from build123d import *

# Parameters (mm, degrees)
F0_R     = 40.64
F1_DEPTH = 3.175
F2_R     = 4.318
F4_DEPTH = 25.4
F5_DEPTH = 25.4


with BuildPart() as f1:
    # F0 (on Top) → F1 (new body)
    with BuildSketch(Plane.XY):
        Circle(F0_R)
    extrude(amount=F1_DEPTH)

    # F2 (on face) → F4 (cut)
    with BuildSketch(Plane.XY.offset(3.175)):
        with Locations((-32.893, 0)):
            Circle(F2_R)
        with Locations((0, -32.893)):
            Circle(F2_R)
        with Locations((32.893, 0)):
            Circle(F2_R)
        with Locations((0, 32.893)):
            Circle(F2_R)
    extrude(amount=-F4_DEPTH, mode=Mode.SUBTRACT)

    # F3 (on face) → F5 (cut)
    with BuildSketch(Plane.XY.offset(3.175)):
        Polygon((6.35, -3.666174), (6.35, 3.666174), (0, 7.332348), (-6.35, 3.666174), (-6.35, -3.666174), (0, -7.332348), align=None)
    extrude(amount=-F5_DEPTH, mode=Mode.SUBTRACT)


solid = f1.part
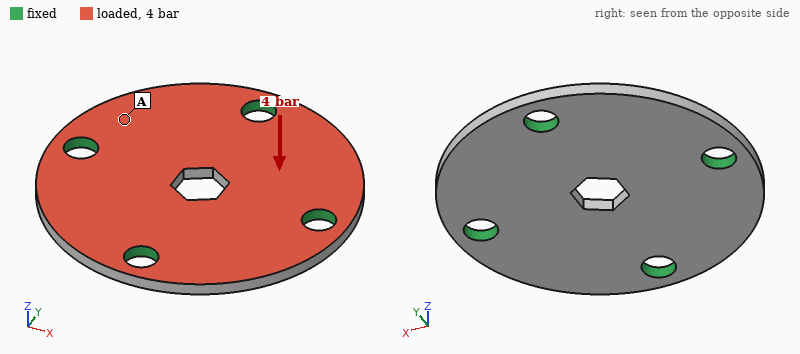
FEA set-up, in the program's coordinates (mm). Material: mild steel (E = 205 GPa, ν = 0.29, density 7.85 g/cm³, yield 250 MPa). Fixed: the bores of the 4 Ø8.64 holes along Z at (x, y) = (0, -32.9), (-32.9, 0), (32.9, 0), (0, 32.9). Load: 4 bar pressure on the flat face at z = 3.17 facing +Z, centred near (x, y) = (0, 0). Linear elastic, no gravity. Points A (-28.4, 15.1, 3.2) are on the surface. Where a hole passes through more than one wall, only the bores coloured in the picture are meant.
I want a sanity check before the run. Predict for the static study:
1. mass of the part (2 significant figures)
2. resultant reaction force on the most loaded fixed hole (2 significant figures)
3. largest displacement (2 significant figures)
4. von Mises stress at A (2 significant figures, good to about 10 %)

120 g
480 N
12 µm
11 MPa
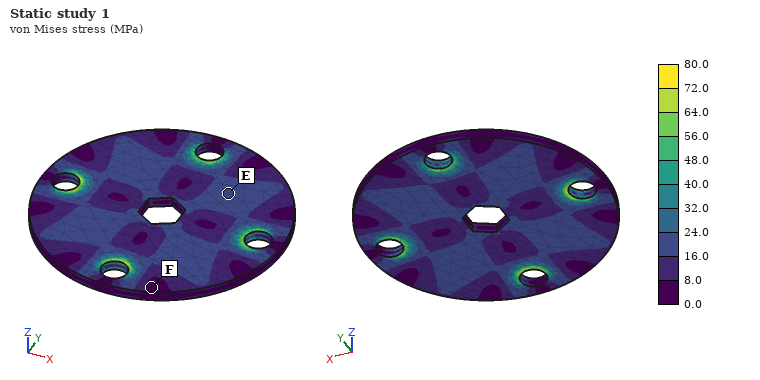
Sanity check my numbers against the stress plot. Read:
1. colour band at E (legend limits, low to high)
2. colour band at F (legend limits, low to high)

16.0 to 24.0 MPa
0.0 to 8.0 MPa
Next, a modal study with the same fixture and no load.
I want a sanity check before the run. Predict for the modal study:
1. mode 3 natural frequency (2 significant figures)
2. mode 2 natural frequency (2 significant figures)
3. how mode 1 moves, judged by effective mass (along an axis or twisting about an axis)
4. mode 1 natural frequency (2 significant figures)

7600 Hz
7400 Hz
along Z
7000 Hz
